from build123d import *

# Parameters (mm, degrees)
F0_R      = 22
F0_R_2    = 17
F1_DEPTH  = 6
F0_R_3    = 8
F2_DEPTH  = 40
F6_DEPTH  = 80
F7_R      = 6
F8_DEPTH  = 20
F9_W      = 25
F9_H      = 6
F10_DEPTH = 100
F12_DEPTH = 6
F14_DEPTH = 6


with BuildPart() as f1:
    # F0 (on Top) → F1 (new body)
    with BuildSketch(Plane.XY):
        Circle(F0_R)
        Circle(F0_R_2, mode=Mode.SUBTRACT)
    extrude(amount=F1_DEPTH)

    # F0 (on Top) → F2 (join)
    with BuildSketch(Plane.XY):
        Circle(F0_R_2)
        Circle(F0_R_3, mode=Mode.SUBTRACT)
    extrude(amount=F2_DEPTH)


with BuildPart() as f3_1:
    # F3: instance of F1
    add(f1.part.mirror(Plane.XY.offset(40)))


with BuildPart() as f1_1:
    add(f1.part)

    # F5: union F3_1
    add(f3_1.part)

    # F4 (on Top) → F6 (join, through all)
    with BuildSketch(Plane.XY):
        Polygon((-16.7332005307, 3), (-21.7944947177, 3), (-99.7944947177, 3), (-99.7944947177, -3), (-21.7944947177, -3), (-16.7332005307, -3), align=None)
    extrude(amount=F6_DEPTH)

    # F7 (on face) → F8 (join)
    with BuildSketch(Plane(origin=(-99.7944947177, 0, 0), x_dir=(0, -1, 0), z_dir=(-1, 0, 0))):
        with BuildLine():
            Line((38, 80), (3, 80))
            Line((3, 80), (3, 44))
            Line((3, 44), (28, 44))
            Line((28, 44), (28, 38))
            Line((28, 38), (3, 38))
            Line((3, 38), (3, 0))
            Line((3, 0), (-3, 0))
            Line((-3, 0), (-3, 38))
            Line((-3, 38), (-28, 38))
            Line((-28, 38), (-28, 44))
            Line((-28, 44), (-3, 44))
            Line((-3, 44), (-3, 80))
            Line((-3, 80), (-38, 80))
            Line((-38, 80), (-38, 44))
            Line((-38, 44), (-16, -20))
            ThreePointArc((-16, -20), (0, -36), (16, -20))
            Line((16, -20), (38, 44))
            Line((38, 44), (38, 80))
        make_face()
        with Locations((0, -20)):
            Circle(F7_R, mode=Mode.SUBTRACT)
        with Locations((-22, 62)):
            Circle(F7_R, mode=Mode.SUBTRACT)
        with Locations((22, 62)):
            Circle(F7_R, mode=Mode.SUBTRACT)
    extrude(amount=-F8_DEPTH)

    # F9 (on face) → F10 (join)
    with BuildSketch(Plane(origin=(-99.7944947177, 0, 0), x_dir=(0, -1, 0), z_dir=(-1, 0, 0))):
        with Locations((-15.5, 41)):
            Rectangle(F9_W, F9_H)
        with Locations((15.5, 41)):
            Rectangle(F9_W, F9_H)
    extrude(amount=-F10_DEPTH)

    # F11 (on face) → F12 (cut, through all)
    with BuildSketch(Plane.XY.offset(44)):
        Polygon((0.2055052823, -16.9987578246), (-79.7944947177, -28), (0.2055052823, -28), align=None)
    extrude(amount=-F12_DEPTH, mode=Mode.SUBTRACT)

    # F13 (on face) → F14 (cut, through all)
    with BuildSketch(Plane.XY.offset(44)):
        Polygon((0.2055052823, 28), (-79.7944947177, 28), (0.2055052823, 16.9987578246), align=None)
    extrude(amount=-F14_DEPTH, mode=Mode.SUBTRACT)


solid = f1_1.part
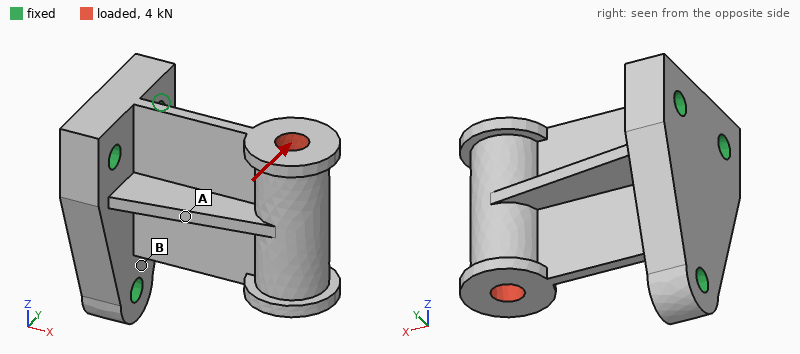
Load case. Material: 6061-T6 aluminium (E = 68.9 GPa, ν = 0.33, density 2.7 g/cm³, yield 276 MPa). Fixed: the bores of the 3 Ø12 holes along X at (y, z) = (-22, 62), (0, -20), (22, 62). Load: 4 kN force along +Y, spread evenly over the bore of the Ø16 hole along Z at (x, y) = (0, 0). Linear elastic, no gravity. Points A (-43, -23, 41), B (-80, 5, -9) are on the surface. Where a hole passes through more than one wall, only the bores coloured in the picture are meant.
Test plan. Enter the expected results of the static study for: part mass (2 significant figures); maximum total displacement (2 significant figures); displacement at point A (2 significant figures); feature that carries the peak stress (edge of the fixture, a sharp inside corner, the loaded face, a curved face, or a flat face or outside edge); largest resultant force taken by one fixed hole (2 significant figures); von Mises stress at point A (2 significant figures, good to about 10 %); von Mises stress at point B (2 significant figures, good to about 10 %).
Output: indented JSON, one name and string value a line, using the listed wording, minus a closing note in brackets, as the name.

{
  "part mass": "640 g",
  "maximum total displacement": "0.37 mm",
  "displacement at point A": "0.10 mm",
  "feature that carries the peak stress": "a flat face or outside edge",
  "largest resultant force taken by one fixed hole": "6.5 kN",
  "von Mises stress at point A": "82 MPa",
  "von Mises stress at point B": "14 MPa"
}
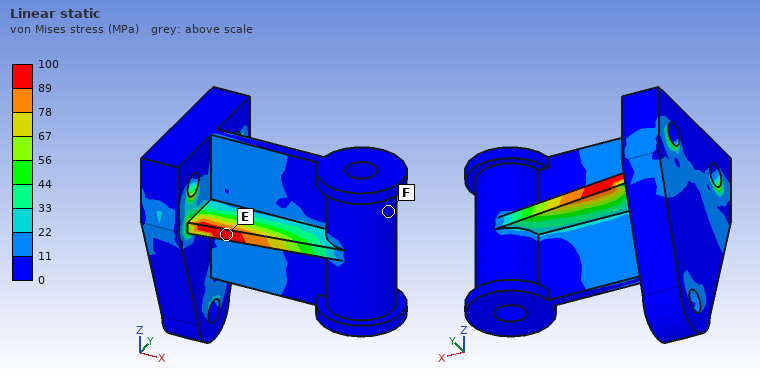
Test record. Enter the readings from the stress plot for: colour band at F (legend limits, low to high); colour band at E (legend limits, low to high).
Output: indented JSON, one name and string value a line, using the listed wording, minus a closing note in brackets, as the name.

{
  "colour band at F": "0 to 11 MPa",
  "colour band at E": "89 to 100 MPa"
}
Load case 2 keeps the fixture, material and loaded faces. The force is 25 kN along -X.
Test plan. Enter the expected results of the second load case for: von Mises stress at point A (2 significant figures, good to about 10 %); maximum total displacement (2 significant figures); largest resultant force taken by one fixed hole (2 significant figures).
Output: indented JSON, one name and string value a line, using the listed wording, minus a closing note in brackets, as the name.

{
  "von Mises stress at point A": "31 MPa",
  "maximum total displacement": "68 µm",
  "largest resultant force taken by one fixed hole": "9.6 kN"
}
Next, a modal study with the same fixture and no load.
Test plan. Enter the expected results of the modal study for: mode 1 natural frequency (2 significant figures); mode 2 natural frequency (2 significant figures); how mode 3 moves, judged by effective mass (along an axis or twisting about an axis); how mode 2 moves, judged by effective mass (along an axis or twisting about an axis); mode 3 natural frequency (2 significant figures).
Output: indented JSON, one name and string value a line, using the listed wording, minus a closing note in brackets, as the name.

{
  "mode 1 natural frequency": "1100 Hz",
  "mode 2 natural frequency": "1400 Hz",
  "how mode 3 moves, judged by effective mass": "along Z",
  "how mode 2 moves, judged by effective mass": "along Y",
  "mode 3 natural frequency": "2300 Hz"
}
